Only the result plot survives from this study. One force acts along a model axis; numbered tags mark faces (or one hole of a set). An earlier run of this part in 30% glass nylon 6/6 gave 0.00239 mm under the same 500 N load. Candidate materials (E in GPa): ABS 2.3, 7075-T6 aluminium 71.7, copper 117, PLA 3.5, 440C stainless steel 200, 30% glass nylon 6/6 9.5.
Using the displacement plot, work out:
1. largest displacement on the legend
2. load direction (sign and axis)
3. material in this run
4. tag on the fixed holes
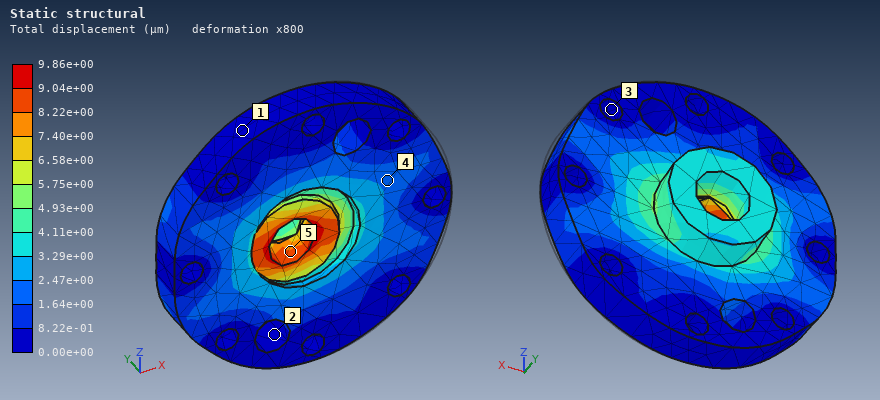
9.86e+00 µm
-X
ABS
3
